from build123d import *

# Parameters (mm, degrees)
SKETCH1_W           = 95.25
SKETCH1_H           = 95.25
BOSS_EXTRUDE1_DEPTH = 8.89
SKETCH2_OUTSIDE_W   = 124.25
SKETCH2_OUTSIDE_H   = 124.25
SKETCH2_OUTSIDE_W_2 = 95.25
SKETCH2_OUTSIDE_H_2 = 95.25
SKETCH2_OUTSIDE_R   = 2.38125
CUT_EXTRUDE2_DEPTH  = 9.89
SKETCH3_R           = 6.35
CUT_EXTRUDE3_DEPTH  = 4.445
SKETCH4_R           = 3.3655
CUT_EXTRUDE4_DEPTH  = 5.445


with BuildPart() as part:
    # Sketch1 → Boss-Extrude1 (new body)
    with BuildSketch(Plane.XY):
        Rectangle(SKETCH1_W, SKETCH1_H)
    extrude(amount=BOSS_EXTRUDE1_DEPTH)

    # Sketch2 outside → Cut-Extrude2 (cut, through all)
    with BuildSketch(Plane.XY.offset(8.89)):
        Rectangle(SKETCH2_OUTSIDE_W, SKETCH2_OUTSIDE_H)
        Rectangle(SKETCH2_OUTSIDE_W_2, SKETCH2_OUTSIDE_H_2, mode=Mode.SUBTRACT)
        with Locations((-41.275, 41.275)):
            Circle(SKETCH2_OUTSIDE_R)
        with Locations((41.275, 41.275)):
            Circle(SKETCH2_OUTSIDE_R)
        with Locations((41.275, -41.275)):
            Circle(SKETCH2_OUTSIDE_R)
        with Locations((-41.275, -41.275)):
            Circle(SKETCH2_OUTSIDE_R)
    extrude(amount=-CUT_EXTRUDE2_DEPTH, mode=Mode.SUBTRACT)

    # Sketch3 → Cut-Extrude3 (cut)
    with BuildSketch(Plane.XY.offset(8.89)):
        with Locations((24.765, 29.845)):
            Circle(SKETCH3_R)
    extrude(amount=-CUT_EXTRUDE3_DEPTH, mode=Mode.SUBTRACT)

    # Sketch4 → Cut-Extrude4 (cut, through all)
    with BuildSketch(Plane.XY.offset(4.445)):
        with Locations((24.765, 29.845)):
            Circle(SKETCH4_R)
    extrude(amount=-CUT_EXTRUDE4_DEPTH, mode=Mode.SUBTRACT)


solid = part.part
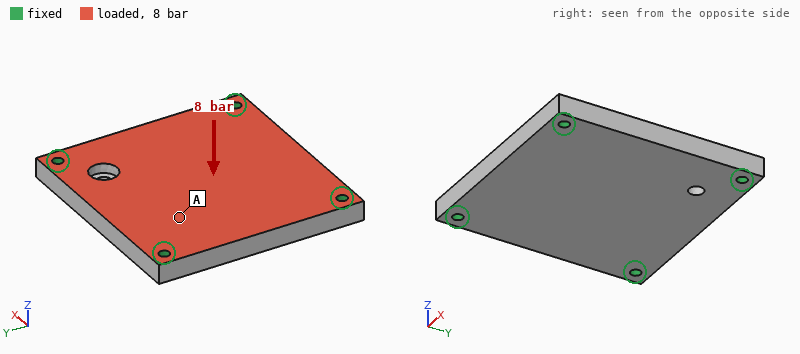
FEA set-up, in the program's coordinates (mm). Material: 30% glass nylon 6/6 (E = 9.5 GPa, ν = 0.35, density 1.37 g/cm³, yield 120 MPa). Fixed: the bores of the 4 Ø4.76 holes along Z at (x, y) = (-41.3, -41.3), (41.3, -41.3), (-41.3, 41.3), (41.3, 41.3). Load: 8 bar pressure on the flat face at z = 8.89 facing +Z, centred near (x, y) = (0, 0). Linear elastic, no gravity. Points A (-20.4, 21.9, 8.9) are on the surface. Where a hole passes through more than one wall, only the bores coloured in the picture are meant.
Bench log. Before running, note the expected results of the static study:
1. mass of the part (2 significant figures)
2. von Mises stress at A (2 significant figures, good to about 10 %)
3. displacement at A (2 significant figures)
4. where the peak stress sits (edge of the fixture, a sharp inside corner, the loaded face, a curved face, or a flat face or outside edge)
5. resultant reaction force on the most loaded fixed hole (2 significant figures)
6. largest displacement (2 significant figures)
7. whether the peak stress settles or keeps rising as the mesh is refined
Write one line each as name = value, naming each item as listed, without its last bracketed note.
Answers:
mass of the part = 110 g
von Mises stress at A = 15 MPa
displacement at A = 0.38 mm
where the peak stress sits = edge of the fixture
resultant reaction force on the most loaded fixed hole = 1.8 kN
largest displacement = 0.55 mm
whether the peak stress settles or keeps rising as the mesh is refined = keeps rising
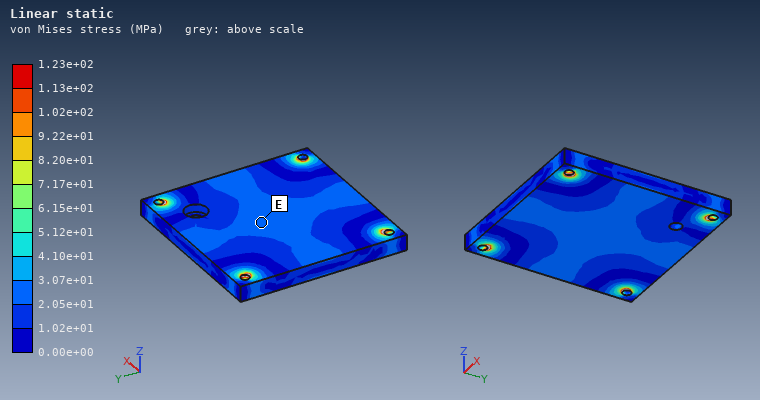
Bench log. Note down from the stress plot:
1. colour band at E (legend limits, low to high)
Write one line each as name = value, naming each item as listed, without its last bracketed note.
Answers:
colour band at E = 2.05e+01 to 3.07e+01 MPa
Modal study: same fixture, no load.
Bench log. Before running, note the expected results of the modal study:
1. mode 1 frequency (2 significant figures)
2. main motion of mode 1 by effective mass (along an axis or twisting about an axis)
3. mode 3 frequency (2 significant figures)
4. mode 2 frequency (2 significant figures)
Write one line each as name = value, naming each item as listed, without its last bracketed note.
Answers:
mode 1 frequency = 2100 Hz
main motion of mode 1 by effective mass = along Z
mode 3 frequency = 3500 Hz
mode 2 frequency = 3500 Hz
